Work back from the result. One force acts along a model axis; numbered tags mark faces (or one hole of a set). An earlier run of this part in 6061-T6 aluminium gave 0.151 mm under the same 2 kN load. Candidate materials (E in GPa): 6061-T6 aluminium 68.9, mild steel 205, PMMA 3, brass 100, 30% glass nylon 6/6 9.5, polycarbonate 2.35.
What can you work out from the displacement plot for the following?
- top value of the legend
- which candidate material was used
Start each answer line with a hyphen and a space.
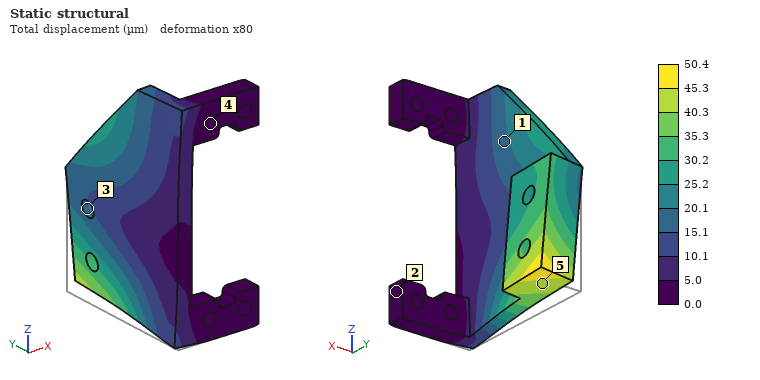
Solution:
- 50.4 µm
- mild steel
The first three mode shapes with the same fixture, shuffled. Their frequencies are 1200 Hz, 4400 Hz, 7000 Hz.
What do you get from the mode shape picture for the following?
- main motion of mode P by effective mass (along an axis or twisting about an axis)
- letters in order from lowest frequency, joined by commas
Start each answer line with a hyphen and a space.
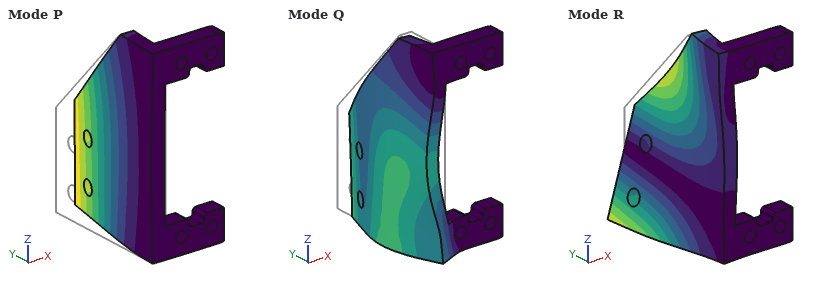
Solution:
- along X
- P, R, Q
